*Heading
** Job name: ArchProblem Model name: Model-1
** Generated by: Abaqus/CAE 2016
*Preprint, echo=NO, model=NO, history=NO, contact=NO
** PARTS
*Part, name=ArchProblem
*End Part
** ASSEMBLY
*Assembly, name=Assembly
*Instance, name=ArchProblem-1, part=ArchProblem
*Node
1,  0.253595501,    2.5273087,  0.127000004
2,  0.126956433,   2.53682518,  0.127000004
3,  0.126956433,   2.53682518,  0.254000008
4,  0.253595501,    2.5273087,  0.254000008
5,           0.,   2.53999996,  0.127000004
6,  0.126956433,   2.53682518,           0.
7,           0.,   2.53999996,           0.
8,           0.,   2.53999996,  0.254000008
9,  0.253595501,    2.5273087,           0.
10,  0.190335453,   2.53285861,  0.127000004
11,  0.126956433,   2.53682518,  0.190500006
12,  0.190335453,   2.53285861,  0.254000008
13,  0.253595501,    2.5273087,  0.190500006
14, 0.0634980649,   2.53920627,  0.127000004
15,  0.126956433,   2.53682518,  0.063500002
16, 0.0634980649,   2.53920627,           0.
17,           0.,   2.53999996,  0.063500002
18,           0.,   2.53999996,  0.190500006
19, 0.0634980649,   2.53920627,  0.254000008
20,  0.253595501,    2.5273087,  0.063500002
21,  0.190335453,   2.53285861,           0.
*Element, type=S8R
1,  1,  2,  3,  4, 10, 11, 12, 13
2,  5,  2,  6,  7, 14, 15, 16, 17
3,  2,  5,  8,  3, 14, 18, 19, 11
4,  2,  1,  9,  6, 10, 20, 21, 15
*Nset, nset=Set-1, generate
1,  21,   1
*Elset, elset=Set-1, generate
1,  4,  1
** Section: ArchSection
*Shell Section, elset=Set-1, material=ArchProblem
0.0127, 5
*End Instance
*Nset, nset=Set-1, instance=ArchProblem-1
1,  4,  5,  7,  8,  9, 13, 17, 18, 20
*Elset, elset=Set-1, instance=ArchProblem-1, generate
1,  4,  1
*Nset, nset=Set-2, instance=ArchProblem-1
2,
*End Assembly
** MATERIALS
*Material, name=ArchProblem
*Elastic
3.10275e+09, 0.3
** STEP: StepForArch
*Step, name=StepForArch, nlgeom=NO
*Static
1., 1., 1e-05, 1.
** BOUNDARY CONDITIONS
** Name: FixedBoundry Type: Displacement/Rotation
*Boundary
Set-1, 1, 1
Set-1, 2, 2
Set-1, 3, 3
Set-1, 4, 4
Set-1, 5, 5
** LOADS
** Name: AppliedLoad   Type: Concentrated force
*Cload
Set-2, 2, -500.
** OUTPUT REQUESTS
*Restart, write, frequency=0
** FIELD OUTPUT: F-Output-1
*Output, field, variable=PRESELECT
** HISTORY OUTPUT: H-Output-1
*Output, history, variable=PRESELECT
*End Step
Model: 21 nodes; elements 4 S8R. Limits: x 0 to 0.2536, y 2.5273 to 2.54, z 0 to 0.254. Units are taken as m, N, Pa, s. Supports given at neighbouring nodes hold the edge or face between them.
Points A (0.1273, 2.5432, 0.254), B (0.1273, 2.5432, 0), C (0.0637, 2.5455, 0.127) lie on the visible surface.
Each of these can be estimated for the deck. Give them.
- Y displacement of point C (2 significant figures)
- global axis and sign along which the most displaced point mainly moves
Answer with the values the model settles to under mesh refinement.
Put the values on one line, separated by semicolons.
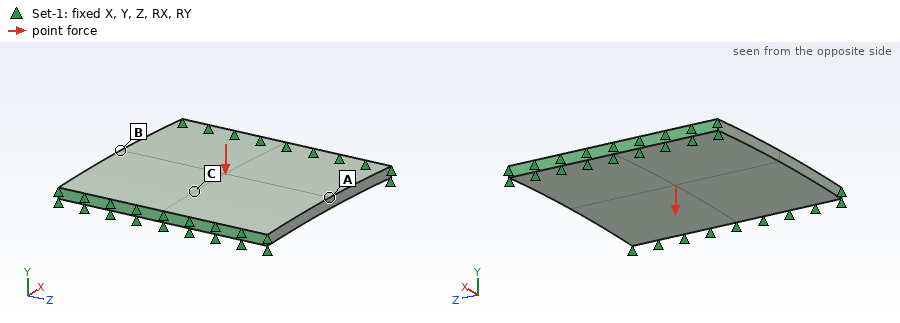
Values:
-3.9e-04 m; -Y
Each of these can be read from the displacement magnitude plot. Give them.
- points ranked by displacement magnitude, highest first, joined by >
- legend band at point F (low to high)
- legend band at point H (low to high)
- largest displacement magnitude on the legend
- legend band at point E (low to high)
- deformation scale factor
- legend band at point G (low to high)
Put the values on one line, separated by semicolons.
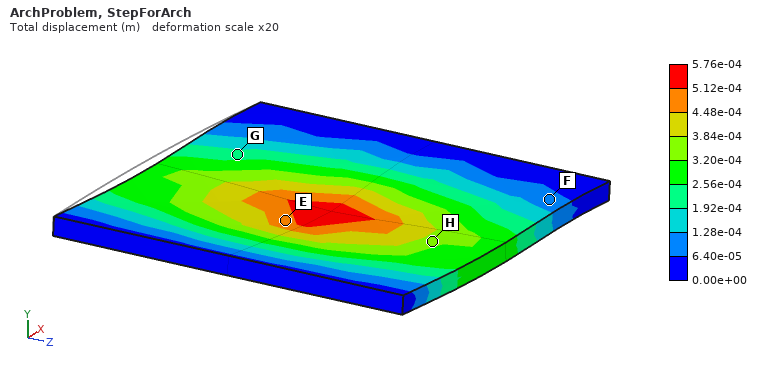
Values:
E > H > G > F; 6.40e-05 to 1.28e-04 m; 3.20e-04 to 3.84e-04 m; 5.76e-04 m; 4.48e-04 to 5.12e-04 m; 20; 1.92e-04 to 2.56e-04 m
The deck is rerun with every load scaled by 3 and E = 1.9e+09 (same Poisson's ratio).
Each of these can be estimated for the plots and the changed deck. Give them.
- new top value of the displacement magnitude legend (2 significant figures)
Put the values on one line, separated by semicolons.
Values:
0.0028 m
